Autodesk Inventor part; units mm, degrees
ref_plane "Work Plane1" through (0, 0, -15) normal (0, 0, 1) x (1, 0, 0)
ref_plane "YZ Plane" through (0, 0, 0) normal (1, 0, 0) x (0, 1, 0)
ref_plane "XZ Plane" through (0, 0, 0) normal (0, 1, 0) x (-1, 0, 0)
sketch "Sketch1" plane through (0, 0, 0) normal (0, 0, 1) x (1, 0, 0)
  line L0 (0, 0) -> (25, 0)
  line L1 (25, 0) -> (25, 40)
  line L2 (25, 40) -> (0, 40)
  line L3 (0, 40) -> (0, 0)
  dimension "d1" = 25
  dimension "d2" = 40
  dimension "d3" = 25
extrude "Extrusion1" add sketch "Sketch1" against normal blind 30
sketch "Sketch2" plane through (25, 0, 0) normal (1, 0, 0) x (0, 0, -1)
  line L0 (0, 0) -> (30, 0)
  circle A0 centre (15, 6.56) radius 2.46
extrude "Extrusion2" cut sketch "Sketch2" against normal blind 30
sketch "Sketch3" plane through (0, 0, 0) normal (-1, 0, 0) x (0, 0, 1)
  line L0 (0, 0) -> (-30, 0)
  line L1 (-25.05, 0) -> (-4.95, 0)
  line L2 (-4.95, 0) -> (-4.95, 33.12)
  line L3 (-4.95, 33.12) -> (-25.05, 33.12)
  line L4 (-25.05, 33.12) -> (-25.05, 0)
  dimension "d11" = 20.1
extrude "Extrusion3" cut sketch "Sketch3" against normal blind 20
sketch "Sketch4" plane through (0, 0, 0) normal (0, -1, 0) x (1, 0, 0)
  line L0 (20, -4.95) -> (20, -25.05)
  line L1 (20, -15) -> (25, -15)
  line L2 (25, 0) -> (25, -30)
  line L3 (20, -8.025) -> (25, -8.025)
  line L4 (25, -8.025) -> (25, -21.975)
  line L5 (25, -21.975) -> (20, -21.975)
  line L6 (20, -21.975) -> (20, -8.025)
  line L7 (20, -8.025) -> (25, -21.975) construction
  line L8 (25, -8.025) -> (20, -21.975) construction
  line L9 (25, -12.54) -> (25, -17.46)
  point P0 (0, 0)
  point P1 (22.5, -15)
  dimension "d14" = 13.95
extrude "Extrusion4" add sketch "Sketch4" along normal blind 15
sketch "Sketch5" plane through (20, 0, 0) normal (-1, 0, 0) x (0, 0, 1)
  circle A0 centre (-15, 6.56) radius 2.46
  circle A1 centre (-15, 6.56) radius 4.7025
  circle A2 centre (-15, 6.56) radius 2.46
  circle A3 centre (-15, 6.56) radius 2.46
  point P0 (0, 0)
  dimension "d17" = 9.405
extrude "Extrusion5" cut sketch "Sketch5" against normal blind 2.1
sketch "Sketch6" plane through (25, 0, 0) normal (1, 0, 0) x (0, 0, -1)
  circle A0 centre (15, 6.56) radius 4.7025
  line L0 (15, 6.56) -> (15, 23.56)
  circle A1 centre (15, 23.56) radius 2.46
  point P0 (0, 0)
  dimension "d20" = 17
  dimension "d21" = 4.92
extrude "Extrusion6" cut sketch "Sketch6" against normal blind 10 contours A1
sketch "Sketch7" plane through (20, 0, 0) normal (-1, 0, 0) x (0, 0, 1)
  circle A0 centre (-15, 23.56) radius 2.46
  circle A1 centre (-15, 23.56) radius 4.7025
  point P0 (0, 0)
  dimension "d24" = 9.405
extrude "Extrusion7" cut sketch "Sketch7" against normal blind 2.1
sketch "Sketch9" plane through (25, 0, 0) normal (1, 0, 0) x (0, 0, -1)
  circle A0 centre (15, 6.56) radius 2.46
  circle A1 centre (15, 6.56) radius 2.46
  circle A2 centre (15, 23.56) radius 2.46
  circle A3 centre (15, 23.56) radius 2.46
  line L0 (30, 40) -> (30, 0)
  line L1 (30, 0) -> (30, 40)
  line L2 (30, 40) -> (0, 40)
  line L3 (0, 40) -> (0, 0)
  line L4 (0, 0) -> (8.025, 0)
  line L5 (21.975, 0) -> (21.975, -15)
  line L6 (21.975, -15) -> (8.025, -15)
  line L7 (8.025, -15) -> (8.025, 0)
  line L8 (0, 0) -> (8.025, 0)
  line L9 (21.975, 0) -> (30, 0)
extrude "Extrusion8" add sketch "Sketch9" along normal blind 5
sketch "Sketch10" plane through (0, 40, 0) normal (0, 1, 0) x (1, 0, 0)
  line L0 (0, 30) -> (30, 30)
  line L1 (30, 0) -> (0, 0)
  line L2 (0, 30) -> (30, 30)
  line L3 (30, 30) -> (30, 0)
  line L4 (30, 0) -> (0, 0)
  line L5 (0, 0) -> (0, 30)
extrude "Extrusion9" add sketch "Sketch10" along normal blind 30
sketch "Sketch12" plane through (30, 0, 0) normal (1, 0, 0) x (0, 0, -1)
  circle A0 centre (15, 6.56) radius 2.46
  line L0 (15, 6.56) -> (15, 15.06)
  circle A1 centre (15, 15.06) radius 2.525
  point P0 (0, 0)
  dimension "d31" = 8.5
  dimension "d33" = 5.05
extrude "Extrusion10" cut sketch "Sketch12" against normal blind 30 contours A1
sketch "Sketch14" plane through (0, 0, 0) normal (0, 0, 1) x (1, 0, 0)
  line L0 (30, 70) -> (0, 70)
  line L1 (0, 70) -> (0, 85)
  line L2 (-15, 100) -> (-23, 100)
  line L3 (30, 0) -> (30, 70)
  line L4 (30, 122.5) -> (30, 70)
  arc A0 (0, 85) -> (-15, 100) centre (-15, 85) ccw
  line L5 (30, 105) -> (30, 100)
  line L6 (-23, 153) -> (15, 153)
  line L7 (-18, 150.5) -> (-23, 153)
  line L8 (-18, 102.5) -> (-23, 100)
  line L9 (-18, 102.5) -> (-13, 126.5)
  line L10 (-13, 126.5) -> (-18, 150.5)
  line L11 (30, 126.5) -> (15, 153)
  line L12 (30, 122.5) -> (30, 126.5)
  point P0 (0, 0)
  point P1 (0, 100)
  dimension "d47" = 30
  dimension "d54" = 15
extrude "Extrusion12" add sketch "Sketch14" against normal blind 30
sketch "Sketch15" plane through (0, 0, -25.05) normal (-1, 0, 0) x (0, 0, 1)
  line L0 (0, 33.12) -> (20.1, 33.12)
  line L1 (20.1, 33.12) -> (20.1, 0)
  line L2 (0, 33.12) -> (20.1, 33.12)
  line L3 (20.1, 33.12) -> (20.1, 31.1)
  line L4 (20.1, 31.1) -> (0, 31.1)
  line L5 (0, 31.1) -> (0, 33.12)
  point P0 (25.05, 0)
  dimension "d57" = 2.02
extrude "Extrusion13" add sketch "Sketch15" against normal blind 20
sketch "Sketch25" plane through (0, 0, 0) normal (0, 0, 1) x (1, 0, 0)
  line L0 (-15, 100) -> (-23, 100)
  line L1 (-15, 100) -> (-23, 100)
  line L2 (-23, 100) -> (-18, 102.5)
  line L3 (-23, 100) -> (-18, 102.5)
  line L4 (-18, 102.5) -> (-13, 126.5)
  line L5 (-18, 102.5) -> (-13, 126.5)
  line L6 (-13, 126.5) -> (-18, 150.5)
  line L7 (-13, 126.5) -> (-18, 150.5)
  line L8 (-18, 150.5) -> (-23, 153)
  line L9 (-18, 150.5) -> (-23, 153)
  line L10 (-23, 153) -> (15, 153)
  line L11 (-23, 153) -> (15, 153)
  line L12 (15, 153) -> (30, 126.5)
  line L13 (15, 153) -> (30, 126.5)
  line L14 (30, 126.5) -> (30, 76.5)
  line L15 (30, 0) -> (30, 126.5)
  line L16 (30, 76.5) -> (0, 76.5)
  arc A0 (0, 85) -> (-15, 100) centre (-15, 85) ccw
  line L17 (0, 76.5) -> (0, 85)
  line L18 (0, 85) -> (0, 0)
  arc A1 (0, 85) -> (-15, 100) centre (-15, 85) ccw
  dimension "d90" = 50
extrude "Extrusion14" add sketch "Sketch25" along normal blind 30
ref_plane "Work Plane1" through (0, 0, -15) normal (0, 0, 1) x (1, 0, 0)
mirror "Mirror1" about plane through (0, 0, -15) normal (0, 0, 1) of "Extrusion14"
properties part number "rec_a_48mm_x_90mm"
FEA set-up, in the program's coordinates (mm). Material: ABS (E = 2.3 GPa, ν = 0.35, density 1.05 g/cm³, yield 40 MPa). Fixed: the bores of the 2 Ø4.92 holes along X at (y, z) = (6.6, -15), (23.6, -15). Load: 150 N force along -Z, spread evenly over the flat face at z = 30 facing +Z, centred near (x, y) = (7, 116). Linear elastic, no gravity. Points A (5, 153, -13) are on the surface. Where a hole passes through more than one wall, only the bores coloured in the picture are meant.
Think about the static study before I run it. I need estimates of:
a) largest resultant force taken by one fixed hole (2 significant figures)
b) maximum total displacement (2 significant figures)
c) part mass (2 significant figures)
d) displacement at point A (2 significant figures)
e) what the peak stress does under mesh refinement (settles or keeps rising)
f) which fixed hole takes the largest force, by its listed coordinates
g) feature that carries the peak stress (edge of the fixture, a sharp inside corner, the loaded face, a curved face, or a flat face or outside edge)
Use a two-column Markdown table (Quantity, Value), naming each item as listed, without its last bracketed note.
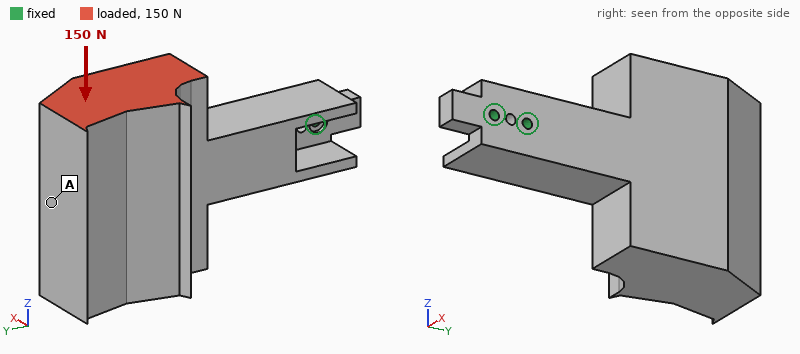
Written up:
| Quantity | Value |
|---|---|
| largest resultant force taken by one fixed hole | 750 N |
| maximum total displacement | 1.3 mm |
| part mass | 340 g |
| displacement at point A | 1.2 mm |
| what the peak stress does under mesh refinement | keeps rising |
| which fixed hole takes the largest force, by its listed coordinates | (23.6, -15) |
| feature that carries the peak stress | edge of the fixture |
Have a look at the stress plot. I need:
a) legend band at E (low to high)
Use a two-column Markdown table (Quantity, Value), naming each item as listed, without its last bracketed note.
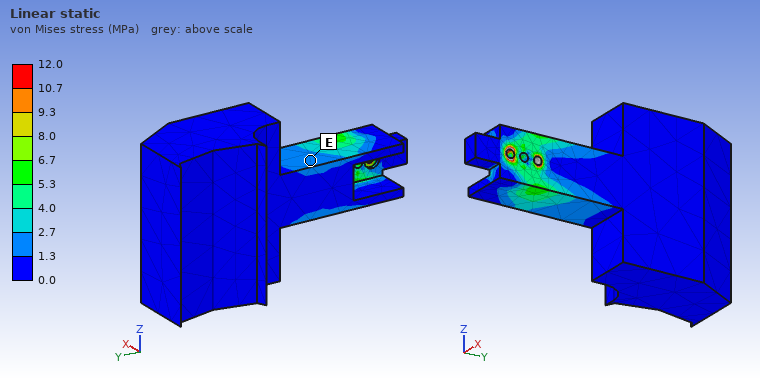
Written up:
| Quantity | Value |
|---|---|
| legend band at E | 1.3 to 2.7 MPa |
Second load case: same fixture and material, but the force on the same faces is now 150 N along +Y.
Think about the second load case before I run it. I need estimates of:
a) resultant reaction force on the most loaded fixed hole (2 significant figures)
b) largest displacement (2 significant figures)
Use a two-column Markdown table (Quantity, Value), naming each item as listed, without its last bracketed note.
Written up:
| Quantity | Value |
|---|---|
| resultant reaction force on the most loaded fixed hole | 320 N |
| largest displacement | 0.77 mm |
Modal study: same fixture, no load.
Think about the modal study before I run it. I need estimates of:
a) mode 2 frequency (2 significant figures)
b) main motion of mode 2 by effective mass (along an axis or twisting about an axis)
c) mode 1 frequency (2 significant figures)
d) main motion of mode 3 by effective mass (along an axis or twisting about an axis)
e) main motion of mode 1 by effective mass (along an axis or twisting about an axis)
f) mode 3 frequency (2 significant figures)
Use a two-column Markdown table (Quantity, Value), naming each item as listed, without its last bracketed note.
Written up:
| Quantity | Value |
|---|---|
| mode 2 frequency | 120 Hz |
| main motion of mode 2 by effective mass | along Z |
| mode 1 frequency | 110 Hz |
| main motion of mode 3 by effective mass | twisting about Y |
| main motion of mode 1 by effective mass | along X |
| mode 3 frequency | 230 Hz |
